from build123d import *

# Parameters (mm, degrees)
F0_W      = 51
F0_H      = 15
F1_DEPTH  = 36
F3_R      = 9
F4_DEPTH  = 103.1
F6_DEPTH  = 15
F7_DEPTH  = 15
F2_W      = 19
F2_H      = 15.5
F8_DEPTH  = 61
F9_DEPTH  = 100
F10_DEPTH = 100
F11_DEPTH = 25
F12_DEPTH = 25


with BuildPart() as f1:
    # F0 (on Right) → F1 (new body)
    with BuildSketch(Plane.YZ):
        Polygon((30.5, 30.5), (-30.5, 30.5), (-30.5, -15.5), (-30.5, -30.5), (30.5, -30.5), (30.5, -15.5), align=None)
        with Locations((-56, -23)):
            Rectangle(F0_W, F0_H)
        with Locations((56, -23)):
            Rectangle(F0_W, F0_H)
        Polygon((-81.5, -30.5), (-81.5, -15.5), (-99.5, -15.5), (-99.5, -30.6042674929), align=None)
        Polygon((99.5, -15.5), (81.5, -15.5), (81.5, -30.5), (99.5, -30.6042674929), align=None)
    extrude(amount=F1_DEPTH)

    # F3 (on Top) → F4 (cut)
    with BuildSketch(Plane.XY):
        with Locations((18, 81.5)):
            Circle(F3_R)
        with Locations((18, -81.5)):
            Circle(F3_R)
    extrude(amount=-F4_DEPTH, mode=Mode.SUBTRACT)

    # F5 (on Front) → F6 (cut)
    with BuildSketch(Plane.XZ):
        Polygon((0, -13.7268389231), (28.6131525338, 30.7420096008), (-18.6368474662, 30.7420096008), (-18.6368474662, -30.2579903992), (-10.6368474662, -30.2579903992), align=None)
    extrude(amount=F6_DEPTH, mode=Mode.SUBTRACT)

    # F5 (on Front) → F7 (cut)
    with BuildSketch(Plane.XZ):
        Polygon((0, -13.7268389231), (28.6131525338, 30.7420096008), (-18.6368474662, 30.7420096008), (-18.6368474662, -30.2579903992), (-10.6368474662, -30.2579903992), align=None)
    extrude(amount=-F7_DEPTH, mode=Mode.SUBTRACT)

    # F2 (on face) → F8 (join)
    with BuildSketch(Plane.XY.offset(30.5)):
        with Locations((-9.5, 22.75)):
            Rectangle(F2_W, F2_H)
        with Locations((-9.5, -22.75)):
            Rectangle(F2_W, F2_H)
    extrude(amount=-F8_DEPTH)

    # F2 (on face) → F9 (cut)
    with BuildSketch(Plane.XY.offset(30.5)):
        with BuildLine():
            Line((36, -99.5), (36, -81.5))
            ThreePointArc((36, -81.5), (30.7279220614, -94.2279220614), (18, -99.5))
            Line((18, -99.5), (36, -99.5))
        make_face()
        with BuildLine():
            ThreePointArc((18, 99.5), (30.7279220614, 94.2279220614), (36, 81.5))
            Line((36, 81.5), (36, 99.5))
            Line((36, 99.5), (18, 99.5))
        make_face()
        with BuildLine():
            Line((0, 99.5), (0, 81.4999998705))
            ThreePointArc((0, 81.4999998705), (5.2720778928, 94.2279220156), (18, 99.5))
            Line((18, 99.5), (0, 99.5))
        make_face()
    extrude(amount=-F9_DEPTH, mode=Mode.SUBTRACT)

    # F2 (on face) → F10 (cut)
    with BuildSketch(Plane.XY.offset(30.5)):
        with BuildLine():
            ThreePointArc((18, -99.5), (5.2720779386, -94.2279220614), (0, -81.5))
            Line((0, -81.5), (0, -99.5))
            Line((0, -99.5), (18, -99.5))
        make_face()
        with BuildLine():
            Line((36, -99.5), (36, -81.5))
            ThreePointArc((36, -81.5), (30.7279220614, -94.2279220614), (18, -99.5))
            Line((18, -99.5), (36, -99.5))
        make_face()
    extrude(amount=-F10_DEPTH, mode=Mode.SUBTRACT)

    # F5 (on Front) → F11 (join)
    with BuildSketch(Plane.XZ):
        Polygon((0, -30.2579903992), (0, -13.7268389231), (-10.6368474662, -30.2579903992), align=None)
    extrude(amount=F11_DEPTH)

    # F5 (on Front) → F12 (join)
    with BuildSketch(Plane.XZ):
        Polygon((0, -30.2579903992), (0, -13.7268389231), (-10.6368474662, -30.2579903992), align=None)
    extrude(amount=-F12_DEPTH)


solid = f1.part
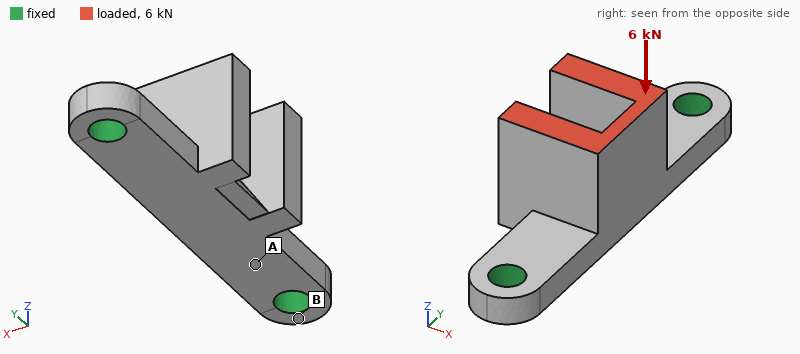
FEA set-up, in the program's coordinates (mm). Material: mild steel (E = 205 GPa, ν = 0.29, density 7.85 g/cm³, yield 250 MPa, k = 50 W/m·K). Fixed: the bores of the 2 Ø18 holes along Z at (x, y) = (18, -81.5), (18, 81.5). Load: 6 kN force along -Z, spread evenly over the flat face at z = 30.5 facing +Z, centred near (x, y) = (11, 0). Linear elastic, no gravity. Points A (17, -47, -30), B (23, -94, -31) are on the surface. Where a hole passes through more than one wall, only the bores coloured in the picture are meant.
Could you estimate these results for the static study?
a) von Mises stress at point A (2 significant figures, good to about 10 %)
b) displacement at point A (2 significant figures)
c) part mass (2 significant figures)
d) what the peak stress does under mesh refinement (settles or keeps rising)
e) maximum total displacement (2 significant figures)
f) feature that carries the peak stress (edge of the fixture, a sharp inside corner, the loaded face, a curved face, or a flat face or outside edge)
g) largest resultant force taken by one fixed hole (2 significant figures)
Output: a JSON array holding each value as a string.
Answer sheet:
["15 MPa", "13 µm", "1.7 kg", "keeps rising", "41 µm", "edge of the fixture", "3.3 kN"]
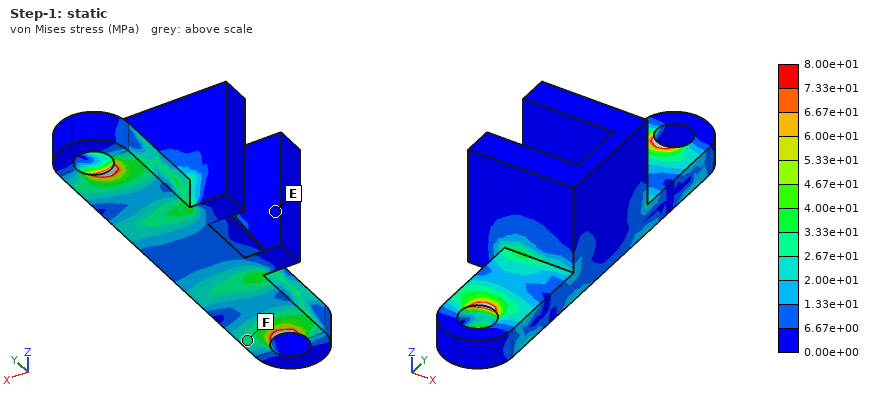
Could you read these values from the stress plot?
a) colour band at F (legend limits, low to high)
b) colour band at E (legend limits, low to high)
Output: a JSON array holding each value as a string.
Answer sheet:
["2.67e+01 to 3.33e+01 MPa", "0.00e+00 to 6.67e+00 MPa"]
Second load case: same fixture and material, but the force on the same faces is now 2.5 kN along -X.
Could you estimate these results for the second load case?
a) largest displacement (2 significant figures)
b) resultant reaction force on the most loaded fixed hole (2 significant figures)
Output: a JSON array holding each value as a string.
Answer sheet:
["86 µm", "1.3 kN"]
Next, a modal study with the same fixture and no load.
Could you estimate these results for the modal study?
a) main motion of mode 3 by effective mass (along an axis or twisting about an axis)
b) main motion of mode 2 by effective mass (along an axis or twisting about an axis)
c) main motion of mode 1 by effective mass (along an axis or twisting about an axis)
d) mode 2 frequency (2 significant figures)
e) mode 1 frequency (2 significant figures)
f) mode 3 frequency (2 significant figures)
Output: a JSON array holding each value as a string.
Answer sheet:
["along Y", "along Z", "along X", "2300 Hz", "1400 Hz", "3600 Hz"]
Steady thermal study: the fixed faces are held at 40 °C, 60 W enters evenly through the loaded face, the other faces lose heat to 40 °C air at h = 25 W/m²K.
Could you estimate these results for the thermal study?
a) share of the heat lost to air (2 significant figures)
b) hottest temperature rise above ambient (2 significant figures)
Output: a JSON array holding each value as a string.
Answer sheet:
["42 %", "59 K"]
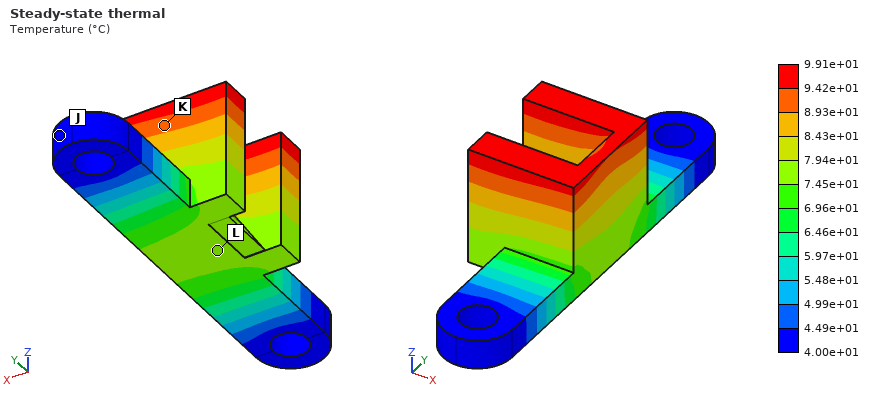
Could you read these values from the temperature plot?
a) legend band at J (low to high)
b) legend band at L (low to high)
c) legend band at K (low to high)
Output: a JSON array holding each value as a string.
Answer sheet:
["4.00e+01 to 4.49e+01 °C", "7.45e+01 to 7.94e+01 °C", "8.93e+01 to 9.42e+01 °C"]
